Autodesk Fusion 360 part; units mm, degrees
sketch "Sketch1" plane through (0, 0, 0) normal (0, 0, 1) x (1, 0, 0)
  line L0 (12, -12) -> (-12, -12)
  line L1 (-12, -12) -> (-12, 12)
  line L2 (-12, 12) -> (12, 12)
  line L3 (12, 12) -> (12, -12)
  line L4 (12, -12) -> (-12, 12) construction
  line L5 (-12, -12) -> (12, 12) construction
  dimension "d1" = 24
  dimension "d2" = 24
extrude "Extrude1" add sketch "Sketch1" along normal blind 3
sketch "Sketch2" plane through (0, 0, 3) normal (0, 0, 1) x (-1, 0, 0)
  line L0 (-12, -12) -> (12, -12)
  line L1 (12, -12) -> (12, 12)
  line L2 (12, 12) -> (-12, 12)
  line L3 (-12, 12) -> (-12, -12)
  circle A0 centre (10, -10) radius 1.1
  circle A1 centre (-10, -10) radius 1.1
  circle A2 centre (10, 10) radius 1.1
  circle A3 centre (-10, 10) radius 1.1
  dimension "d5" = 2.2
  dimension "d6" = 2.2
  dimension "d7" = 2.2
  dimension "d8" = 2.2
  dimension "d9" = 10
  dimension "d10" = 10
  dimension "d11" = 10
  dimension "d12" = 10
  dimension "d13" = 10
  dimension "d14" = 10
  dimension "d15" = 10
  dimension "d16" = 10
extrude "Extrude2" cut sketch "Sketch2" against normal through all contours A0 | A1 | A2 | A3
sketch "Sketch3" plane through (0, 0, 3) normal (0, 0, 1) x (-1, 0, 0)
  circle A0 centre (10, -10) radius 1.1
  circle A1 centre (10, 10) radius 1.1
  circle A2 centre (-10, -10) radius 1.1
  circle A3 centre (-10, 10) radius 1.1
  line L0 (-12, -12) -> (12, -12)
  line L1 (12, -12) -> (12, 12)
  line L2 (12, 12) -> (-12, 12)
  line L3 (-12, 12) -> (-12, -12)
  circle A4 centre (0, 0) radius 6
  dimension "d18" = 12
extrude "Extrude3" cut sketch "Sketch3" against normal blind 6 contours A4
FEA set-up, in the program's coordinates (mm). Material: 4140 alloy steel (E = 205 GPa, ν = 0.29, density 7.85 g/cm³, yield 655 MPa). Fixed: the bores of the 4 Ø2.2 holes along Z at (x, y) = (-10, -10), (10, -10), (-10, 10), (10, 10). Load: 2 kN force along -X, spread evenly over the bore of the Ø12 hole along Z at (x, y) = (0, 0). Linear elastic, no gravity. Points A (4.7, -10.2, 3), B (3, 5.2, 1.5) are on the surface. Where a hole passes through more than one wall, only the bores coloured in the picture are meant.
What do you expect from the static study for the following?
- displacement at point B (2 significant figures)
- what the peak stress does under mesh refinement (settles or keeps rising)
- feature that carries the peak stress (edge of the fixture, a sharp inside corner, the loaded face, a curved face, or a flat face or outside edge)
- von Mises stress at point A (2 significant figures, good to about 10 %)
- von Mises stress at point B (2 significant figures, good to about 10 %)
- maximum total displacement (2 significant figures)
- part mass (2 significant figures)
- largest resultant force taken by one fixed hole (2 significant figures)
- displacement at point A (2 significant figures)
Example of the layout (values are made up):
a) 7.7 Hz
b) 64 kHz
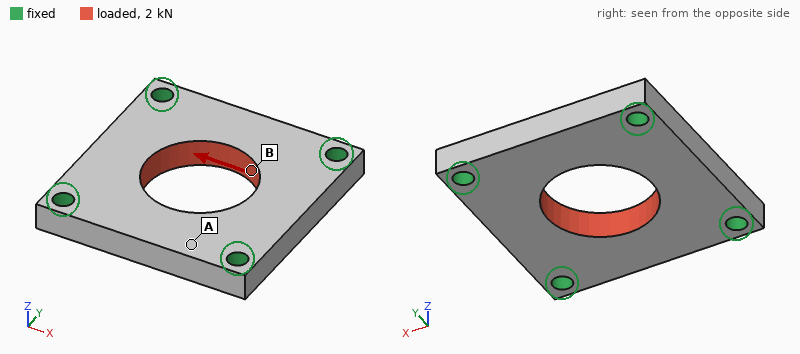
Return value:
a) 1.4 µm
b) keeps rising
c) edge of the fixture
d) 19 MPa
e) 42 MPa
f) 2.3 µm
g) 11 g
h) 540 N
i) 0.57 µm
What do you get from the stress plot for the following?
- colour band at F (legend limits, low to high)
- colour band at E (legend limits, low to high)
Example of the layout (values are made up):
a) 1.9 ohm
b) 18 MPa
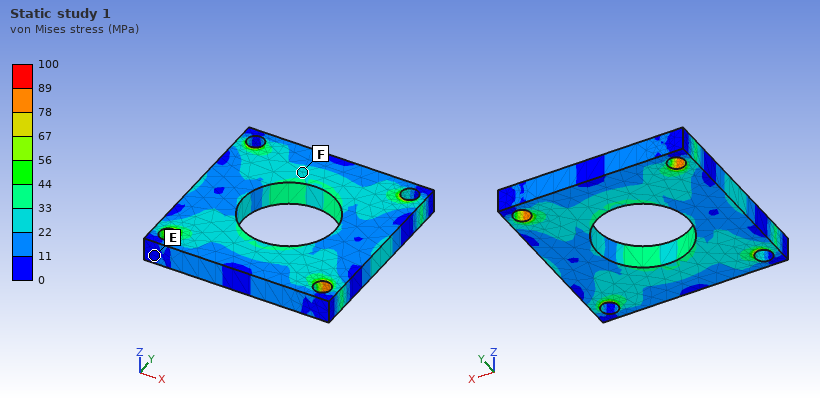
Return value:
a) 22 to 33 MPa
b) 0 to 11 MPa
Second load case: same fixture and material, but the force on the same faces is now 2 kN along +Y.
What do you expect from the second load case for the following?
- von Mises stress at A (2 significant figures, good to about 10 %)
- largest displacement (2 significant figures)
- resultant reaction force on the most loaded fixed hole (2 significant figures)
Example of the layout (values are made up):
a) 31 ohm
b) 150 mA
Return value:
a) 16 MPa
b) 2.3 µm
c) 540 N
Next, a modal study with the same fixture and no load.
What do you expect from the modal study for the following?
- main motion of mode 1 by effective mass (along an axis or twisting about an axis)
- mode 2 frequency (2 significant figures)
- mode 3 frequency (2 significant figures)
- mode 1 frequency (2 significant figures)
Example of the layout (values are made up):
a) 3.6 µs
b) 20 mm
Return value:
a) along Z
b) 38 kHz
c) 38 kHz
d) 30 kHz
